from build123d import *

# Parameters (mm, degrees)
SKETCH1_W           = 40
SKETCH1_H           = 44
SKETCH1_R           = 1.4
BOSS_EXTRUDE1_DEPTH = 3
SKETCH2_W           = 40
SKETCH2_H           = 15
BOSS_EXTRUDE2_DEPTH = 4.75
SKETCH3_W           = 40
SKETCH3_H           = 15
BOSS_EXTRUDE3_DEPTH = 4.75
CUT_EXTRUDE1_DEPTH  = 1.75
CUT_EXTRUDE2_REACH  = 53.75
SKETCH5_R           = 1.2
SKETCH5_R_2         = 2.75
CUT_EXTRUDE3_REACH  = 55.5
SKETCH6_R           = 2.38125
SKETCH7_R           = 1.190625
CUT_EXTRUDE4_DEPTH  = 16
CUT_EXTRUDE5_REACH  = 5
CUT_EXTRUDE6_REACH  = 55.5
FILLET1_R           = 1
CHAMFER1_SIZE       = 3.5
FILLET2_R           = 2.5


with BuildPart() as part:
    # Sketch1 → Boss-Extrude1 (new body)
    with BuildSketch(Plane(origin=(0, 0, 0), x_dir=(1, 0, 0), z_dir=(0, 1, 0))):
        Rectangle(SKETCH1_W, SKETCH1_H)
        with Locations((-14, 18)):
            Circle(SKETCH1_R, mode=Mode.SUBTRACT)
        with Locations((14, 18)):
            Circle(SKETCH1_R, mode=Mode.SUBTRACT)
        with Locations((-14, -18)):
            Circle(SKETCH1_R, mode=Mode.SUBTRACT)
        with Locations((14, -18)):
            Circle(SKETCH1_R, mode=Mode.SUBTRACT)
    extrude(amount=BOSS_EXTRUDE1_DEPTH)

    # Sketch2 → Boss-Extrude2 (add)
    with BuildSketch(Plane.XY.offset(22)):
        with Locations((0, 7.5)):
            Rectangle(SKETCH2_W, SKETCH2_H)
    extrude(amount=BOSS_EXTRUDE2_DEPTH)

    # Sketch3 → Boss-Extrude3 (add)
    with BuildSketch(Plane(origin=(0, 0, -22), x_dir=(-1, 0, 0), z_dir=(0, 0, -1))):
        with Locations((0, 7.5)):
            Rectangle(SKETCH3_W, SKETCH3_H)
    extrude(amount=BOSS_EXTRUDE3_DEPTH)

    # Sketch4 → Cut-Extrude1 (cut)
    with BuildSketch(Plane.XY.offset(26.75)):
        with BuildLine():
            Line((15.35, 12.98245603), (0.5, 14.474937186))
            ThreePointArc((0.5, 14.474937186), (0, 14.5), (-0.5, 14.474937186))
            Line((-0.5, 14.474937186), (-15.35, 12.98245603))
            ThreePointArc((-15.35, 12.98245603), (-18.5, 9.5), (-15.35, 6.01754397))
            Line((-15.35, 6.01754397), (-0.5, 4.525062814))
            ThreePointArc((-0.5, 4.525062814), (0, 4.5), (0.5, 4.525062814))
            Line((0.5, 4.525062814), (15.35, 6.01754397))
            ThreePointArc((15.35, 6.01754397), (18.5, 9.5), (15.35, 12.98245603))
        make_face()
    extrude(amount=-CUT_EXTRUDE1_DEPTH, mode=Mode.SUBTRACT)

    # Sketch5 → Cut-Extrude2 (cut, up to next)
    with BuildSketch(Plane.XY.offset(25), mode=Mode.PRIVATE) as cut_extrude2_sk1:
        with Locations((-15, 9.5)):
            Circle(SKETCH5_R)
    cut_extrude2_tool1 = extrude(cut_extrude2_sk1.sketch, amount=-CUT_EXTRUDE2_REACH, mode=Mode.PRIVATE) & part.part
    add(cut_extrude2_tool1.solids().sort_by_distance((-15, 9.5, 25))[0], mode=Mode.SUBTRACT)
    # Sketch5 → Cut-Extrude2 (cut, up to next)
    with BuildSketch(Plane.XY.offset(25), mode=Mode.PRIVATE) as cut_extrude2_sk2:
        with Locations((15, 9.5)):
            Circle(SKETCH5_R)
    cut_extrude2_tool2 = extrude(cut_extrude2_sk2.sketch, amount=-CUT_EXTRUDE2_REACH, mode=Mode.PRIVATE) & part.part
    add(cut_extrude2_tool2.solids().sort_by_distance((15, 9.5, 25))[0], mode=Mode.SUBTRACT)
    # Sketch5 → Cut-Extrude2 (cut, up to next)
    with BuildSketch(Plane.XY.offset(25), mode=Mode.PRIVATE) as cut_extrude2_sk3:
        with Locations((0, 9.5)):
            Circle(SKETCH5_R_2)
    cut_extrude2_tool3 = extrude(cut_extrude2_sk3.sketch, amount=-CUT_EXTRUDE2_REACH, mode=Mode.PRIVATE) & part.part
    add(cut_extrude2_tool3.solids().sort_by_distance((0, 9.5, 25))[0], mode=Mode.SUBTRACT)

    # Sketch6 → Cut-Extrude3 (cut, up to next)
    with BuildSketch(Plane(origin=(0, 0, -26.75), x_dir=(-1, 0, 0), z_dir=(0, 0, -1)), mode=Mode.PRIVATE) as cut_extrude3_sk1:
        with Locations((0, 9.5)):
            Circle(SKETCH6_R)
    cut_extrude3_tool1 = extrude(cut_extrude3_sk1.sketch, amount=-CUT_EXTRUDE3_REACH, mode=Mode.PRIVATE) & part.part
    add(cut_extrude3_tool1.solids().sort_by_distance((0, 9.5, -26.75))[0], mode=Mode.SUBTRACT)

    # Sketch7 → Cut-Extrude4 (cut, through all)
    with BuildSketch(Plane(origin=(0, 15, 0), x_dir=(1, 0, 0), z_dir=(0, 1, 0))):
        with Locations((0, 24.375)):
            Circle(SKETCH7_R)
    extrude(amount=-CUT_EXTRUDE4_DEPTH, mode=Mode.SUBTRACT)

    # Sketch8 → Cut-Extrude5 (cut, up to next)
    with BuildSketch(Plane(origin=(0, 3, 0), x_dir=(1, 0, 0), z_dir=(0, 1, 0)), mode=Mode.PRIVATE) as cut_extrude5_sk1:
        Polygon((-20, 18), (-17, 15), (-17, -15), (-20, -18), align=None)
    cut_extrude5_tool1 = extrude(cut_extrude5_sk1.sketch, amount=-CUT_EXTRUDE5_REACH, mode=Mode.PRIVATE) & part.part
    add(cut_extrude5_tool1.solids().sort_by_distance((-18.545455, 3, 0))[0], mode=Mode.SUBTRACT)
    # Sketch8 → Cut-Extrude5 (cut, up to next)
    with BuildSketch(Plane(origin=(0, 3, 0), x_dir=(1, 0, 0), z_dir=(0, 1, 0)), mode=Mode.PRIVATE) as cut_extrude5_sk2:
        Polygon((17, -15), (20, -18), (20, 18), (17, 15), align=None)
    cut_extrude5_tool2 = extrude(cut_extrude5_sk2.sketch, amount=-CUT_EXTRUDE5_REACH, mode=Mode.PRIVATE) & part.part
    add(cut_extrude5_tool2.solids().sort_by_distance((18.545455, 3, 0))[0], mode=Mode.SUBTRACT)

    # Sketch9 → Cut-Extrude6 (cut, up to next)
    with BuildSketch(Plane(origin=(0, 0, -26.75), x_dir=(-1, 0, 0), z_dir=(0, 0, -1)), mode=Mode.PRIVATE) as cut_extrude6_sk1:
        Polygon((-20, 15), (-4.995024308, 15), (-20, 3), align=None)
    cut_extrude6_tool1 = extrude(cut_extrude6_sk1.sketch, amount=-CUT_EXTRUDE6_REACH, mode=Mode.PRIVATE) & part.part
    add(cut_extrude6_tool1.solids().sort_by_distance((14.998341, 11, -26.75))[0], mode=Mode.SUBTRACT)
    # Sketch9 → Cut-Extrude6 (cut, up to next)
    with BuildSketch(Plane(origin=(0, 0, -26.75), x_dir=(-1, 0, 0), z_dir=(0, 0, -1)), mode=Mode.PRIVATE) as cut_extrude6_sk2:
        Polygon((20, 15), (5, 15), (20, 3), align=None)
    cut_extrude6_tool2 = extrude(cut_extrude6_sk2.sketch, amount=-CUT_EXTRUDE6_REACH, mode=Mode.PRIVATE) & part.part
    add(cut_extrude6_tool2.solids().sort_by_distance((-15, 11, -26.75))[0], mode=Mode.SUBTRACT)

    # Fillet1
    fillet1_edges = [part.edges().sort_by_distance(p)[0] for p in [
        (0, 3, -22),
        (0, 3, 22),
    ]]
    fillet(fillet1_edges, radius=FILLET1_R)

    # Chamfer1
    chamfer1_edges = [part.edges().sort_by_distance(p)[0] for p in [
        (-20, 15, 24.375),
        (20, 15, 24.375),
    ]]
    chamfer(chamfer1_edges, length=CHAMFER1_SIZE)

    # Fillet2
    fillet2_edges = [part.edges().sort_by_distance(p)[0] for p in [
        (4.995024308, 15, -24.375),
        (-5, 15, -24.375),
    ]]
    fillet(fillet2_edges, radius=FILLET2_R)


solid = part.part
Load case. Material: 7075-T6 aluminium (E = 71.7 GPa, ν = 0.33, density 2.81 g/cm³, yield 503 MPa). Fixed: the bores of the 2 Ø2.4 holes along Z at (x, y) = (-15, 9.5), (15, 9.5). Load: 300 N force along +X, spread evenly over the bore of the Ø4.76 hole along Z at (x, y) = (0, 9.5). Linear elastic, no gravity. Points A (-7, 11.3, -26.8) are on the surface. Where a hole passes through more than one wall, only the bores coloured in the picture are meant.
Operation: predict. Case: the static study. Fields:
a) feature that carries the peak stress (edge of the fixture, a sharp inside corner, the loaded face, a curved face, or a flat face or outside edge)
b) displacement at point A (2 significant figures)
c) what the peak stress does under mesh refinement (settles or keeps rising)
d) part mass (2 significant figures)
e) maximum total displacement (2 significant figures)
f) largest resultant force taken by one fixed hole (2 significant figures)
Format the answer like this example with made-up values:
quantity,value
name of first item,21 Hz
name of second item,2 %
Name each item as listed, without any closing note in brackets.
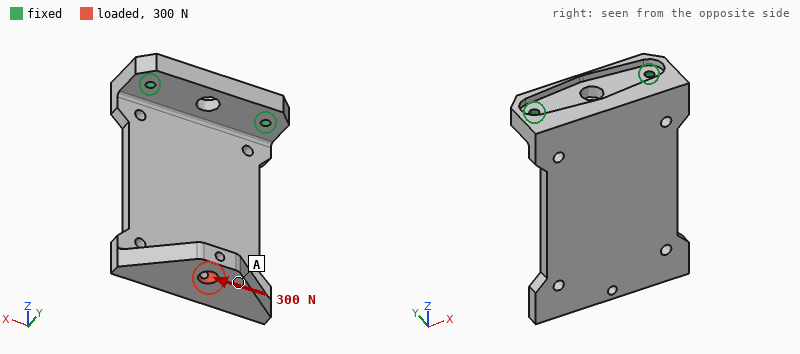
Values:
quantity,value
feature that carries the peak stress,edge of the fixture
displacement at point A,0.24 mm
what the peak stress does under mesh refinement,keeps rising
part mass,24 g
maximum total displacement,0.28 mm
largest resultant force taken by one fixed hole,480 N
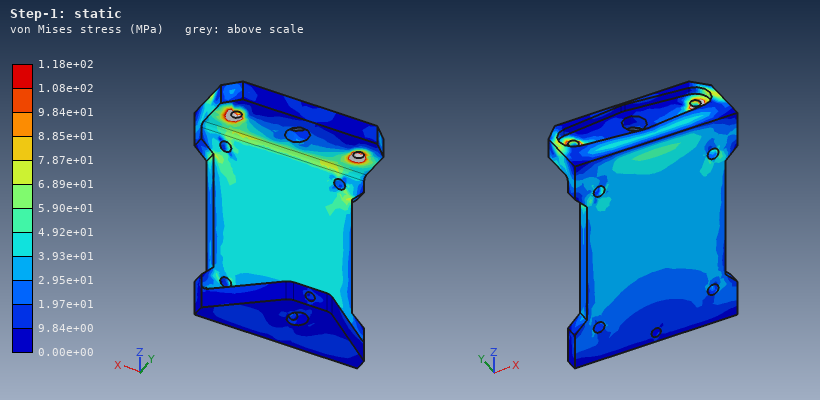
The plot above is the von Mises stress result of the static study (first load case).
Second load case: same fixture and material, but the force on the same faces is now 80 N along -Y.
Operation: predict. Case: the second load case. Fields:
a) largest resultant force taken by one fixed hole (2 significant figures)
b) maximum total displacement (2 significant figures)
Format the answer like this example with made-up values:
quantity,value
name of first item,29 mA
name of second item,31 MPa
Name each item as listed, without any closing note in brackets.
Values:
quantity,value
largest resultant force taken by one fixed hole,40 N
maximum total displacement,0.77 mm
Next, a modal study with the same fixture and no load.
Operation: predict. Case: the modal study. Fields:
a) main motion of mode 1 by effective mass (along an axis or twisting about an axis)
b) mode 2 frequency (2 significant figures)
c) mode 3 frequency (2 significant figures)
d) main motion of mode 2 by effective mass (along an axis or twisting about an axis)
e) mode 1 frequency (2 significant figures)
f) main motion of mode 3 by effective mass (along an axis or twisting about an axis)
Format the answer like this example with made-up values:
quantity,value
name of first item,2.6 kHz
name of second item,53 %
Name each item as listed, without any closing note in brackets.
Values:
quantity,value
main motion of mode 1 by effective mass,along Y
mode 2 frequency,2000 Hz
mode 3 frequency,3300 Hz
main motion of mode 2 by effective mass,along X
mode 1 frequency,590 Hz
main motion of mode 3 by effective mass,along X
